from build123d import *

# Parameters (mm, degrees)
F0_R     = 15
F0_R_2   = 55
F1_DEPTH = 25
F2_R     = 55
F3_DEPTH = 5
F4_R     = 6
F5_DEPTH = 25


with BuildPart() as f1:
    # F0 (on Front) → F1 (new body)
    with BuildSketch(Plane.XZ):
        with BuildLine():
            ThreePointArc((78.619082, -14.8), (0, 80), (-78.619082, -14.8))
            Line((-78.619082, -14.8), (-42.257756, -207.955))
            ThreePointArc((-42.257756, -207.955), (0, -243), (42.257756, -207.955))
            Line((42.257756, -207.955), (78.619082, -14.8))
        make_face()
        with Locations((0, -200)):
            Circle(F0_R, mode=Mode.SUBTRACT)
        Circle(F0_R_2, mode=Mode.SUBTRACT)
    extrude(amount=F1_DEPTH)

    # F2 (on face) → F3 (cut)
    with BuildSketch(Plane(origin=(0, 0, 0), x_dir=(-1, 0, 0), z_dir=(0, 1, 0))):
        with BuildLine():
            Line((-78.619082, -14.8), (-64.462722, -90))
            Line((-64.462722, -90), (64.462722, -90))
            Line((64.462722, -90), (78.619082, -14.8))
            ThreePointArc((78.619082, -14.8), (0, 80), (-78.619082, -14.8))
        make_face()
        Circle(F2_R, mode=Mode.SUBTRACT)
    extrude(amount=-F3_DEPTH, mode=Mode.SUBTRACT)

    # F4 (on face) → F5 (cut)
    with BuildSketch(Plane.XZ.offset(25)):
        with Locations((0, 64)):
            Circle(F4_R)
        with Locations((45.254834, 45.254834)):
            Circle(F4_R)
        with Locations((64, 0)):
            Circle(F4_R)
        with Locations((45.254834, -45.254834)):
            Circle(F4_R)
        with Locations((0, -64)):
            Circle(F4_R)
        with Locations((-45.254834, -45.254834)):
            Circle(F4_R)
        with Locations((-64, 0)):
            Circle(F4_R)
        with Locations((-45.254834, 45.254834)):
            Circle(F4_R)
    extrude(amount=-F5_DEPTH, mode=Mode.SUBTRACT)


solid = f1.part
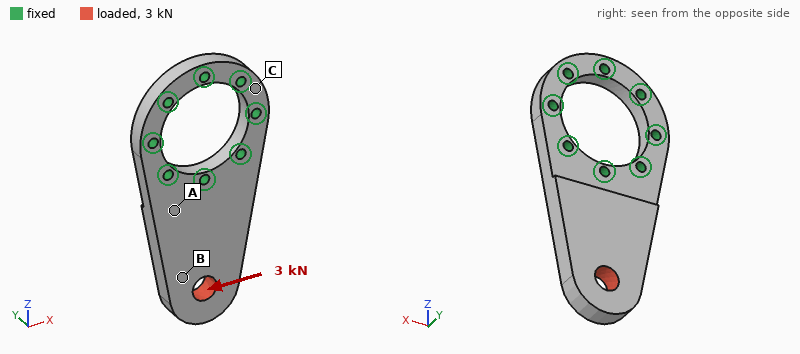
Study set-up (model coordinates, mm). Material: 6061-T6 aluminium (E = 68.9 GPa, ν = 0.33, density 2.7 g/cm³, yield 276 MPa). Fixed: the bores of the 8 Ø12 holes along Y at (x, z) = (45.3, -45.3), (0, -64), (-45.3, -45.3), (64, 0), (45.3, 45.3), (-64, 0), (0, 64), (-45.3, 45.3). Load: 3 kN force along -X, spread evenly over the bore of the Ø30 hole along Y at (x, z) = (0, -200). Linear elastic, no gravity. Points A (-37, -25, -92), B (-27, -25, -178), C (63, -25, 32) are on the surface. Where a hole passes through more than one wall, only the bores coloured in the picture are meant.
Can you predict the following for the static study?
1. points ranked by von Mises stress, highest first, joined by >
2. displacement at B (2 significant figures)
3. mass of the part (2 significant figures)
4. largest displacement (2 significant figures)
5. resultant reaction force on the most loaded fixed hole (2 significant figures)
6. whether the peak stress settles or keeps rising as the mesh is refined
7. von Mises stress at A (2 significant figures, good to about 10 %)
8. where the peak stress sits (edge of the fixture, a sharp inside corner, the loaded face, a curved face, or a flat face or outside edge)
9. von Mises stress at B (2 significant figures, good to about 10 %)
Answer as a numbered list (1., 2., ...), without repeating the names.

1. A > B > C
2. 18 µm
3. 1.6 kg
4. 30 µm
5. 3.4 kN
6. keeps rising
7. 3.8 MPa
8. edge of the fixture
9. 2.0 MPa
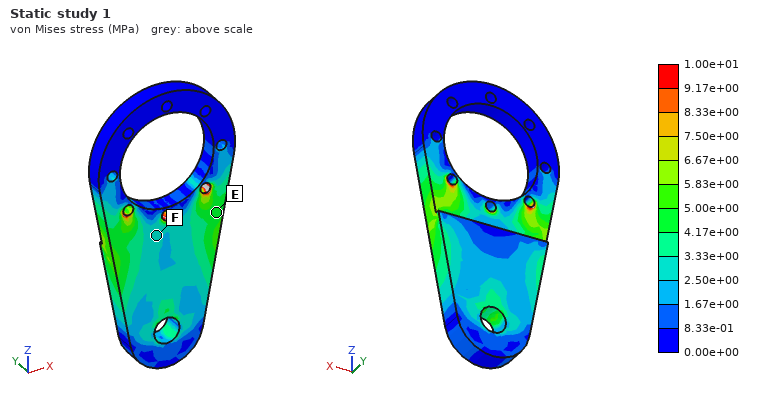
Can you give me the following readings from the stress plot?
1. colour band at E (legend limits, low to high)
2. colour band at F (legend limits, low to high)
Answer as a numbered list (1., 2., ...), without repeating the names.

1. 4.17e+00 to 5.00e+00 MPa
2. 2.50e+00 to 3.33e+00 MPa
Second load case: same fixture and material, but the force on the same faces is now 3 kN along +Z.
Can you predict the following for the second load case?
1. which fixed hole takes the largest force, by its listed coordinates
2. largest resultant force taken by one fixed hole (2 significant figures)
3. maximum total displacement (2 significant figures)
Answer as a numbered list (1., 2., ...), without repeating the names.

1. (0, -64)
2. 1.2 kN
3. 8.5 µm
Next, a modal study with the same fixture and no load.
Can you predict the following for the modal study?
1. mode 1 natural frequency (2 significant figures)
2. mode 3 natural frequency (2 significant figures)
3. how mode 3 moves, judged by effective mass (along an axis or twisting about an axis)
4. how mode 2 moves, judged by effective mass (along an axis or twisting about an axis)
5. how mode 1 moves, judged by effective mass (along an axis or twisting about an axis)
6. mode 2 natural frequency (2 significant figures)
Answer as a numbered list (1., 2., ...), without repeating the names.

1. 640 Hz
2. 2600 Hz
3. along X
4. twisting about Z
5. along Y
6. 2300 Hz
